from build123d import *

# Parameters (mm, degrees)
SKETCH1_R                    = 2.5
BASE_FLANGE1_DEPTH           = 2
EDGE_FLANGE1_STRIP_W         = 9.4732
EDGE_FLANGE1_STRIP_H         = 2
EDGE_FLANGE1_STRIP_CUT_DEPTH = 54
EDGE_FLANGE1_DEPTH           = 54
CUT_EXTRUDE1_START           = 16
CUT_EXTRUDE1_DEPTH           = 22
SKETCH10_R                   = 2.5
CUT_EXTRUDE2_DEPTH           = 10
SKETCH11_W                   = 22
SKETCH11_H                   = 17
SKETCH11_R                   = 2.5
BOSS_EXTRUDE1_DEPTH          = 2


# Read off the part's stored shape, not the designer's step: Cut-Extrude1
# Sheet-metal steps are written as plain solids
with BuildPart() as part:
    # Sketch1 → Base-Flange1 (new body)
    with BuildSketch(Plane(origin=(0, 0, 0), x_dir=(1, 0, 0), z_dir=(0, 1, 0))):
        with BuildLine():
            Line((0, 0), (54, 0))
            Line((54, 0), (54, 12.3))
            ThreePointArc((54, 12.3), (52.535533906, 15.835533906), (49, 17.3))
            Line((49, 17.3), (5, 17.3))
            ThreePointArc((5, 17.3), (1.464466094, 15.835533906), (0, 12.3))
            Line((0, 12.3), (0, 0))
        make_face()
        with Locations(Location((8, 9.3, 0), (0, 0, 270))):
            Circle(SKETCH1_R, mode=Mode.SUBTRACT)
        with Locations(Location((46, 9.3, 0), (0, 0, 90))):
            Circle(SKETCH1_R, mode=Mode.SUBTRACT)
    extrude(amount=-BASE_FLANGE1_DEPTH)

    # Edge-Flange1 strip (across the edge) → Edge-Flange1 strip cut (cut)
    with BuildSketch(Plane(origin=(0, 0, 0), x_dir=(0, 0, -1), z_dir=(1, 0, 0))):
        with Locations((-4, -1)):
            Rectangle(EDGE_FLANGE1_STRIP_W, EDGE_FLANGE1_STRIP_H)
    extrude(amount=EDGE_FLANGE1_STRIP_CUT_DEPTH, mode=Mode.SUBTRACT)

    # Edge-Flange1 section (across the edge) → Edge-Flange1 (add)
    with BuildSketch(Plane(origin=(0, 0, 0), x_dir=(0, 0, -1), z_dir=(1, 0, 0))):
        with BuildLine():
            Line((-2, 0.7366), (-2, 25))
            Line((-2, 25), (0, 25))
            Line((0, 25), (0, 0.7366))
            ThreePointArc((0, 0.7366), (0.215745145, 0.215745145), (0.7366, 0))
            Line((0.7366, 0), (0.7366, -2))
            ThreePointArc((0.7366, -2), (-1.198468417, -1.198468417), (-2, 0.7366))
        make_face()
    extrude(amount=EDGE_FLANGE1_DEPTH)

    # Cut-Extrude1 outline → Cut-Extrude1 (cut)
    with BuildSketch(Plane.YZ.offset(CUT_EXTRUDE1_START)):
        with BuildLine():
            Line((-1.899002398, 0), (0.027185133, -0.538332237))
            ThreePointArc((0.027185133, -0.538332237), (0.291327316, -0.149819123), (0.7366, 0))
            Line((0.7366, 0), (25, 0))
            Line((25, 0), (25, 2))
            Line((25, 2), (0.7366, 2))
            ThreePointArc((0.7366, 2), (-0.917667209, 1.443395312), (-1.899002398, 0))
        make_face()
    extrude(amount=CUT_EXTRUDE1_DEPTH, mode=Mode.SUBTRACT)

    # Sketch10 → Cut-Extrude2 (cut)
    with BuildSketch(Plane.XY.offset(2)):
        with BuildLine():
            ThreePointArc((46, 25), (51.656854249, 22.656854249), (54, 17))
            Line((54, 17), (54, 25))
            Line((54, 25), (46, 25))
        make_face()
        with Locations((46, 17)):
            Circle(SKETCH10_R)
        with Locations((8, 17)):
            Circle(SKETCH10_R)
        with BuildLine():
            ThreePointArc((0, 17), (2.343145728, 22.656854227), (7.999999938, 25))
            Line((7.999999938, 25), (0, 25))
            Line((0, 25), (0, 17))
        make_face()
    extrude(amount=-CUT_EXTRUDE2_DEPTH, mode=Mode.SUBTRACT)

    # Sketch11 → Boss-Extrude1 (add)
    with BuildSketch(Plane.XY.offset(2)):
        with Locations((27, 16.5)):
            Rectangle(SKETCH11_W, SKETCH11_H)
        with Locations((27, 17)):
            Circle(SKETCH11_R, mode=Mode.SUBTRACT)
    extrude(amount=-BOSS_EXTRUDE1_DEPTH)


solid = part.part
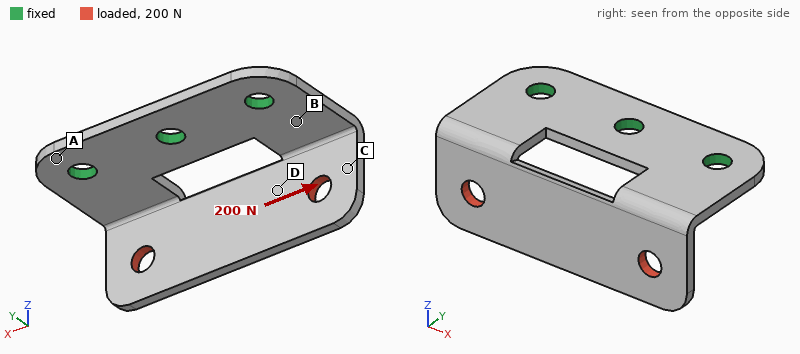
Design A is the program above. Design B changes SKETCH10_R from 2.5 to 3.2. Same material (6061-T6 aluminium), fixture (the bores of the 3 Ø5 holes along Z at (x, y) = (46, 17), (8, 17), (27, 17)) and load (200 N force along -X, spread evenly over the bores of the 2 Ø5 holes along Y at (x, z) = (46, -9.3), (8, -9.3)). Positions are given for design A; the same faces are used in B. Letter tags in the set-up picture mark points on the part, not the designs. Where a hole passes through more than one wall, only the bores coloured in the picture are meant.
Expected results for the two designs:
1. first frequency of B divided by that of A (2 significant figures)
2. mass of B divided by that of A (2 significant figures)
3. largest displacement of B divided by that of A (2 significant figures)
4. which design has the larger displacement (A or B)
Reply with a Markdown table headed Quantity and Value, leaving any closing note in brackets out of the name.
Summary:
| Quantity | Value |
|---|---|
| first frequency of B divided by that of A | 1.0 |
| mass of B divided by that of A | 0.99 |
| largest displacement of B divided by that of A | 0.91 |
| which design has the larger displacement | A |
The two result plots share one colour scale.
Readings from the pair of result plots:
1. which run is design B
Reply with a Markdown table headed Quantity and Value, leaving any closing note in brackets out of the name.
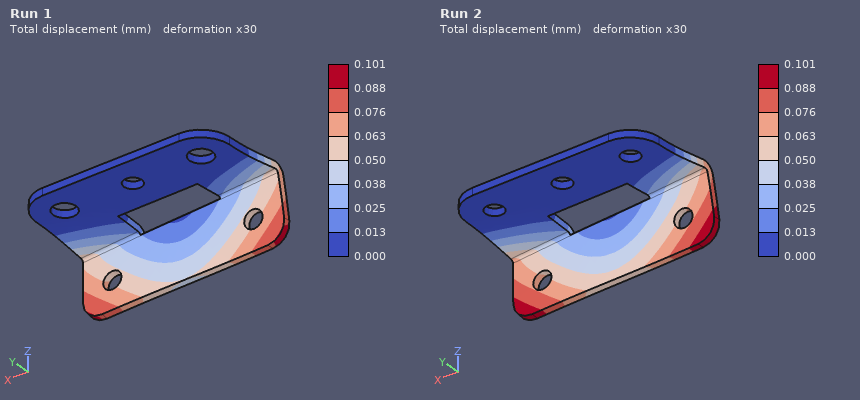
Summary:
| Quantity | Value |
|---|---|
| which run is design B | Run 1 |
